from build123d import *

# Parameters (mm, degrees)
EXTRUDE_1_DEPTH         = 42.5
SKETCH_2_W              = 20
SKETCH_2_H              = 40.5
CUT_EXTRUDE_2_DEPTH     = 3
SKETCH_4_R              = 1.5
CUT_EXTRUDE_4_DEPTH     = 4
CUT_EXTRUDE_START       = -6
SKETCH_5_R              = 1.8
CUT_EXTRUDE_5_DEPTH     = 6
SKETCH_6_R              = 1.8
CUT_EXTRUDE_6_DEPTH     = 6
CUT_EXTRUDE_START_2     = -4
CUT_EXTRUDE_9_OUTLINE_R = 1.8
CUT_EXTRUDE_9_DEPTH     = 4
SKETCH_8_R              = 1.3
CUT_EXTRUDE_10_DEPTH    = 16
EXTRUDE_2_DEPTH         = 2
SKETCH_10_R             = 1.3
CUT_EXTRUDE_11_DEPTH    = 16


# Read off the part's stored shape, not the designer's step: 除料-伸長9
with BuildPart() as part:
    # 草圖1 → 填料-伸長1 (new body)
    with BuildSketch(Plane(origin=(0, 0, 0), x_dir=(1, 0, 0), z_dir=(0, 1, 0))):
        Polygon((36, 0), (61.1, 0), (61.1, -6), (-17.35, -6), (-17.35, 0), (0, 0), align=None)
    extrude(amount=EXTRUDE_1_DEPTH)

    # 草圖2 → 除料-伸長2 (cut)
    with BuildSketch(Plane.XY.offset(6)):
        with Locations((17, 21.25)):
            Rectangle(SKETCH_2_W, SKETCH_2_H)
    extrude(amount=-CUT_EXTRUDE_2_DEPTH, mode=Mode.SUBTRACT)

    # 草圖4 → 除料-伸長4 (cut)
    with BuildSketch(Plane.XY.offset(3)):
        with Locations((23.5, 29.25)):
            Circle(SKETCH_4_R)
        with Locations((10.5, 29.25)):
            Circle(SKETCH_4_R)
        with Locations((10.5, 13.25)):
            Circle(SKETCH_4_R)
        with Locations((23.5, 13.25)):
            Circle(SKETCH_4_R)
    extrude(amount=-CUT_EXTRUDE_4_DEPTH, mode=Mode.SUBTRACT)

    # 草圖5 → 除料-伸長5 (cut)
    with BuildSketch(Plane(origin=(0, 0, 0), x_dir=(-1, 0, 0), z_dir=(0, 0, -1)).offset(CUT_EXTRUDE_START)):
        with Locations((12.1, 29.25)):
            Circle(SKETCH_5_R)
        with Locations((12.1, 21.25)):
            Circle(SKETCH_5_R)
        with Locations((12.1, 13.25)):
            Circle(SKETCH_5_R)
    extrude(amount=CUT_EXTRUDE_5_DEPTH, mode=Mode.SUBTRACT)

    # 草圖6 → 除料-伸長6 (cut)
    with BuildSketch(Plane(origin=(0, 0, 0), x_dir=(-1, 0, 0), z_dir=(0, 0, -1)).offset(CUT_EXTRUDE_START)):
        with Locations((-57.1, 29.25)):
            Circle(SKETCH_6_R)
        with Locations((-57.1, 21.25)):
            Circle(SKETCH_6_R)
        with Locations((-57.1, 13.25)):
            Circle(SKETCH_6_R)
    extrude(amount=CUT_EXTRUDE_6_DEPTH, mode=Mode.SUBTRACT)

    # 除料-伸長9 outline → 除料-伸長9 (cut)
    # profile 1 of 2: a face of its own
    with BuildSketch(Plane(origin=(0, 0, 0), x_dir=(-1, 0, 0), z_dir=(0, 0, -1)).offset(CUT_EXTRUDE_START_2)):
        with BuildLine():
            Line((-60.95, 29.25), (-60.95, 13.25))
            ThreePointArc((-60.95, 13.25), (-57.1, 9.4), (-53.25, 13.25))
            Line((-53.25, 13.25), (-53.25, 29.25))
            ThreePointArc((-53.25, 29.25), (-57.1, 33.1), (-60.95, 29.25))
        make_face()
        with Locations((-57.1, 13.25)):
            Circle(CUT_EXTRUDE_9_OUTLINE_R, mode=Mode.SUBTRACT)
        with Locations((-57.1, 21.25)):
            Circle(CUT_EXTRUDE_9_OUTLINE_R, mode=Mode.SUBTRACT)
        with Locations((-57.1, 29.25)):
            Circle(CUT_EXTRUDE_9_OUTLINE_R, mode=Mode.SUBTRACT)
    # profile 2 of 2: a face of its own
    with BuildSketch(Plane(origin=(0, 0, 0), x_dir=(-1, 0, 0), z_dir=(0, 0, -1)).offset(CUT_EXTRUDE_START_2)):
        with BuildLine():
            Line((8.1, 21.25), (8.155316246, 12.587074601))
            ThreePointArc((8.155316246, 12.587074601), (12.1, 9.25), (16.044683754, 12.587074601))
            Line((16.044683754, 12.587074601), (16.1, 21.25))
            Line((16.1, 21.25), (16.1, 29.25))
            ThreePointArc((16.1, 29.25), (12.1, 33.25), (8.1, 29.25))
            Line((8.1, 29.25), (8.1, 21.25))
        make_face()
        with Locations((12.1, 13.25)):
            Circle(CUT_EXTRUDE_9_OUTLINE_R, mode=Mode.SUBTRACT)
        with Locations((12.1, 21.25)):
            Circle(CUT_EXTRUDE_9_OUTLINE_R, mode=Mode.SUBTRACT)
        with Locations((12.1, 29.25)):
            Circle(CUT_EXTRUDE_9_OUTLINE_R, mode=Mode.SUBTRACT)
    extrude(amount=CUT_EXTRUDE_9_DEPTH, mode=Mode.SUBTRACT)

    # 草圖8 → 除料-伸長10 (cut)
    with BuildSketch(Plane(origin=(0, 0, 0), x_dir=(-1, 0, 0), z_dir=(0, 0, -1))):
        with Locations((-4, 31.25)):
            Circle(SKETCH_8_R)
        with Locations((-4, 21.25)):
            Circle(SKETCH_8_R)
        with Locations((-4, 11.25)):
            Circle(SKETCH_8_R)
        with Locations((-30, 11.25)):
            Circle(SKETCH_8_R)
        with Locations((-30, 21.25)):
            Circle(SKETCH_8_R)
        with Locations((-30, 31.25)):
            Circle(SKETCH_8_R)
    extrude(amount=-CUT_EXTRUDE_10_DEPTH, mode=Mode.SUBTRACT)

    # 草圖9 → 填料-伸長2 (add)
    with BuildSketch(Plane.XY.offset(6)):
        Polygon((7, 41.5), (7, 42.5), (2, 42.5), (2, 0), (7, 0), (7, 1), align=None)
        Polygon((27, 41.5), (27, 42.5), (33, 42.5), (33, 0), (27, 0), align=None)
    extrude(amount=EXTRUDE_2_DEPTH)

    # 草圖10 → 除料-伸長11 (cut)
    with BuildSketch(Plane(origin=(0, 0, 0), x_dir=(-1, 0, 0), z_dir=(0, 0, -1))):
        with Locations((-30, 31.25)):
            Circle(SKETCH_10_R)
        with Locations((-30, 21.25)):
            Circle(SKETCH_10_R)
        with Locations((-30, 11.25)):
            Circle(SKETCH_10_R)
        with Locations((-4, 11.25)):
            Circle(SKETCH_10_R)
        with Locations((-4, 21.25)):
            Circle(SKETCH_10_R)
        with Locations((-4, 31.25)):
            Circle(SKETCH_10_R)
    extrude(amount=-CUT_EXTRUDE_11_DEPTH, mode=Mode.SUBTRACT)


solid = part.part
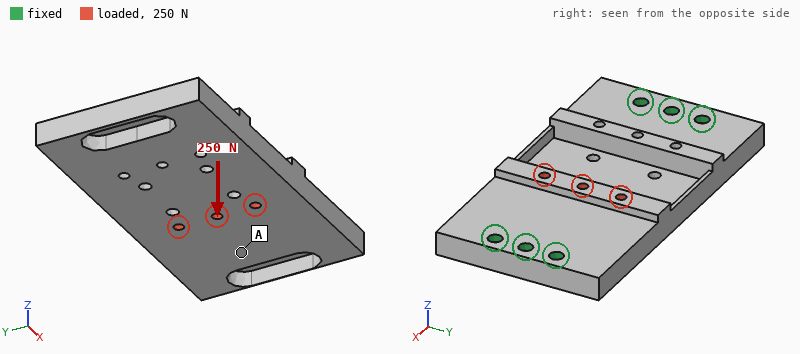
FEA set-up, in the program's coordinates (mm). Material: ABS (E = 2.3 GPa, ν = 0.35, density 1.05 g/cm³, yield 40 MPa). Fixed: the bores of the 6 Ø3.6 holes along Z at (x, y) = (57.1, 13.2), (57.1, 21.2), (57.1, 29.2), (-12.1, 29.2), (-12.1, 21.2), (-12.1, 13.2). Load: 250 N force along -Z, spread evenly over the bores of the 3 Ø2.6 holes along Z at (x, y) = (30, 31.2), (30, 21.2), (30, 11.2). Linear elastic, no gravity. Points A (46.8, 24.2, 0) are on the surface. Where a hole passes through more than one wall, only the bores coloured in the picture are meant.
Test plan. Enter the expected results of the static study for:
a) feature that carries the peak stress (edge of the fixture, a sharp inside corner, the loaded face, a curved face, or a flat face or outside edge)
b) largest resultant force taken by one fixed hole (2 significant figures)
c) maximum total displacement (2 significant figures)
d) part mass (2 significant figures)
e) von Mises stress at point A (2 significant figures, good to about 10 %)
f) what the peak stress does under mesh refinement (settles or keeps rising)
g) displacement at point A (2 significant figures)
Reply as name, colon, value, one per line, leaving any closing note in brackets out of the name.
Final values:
feature that carries the peak stress: edge of the fixture
largest resultant force taken by one fixed hole: 170 N
maximum total displacement: 0.65 mm
part mass: 17 g
von Mises stress at point A: 2.9 MPa
what the peak stress does under mesh refinement: keeps rising
displacement at point A: 0.23 mm
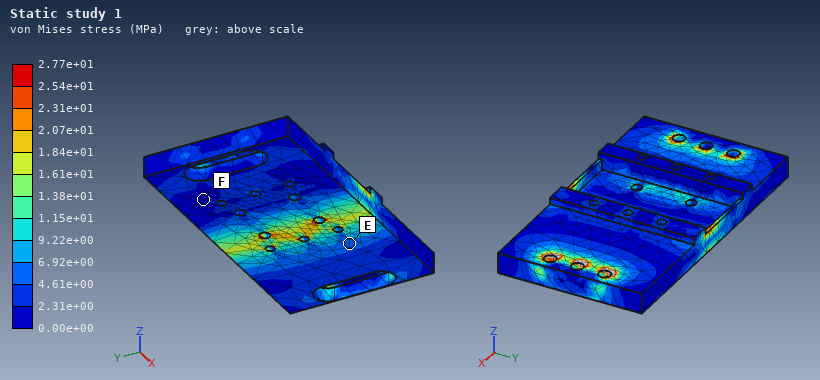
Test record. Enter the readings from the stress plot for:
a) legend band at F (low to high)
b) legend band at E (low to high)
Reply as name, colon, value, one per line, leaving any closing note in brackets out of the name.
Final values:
legend band at F: 0.00e+00 to 2.31e+00 MPa
legend band at E: 4.61e+00 to 6.92e+00 MPa
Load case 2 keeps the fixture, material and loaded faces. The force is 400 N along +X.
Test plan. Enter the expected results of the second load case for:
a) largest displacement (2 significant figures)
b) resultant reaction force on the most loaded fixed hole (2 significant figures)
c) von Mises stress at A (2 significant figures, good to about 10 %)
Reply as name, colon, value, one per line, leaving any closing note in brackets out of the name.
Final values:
largest displacement: 67 µm
resultant reaction force on the most loaded fixed hole: 110 N
von Mises stress at A: 0.71 MPa
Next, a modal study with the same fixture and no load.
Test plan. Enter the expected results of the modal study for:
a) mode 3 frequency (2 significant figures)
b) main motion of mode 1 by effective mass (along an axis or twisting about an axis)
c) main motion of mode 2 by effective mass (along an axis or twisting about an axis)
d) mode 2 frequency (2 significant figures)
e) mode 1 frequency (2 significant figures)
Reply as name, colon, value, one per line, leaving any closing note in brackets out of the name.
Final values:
mode 3 frequency: 2700 Hz
main motion of mode 1 by effective mass: along Z
main motion of mode 2 by effective mass: twisting about X
mode 2 frequency: 1600 Hz
mode 1 frequency: 1300 Hz
